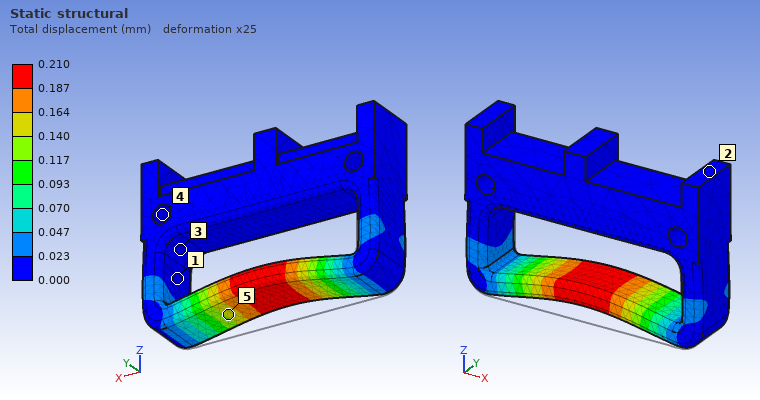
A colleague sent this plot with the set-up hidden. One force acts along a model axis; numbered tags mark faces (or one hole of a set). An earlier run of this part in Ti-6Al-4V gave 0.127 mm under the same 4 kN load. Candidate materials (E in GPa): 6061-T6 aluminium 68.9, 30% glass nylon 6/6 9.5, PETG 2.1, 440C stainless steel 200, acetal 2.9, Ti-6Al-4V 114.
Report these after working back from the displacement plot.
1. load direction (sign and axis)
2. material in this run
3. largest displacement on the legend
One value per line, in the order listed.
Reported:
+Z
6061-T6 aluminium
0.210 mm
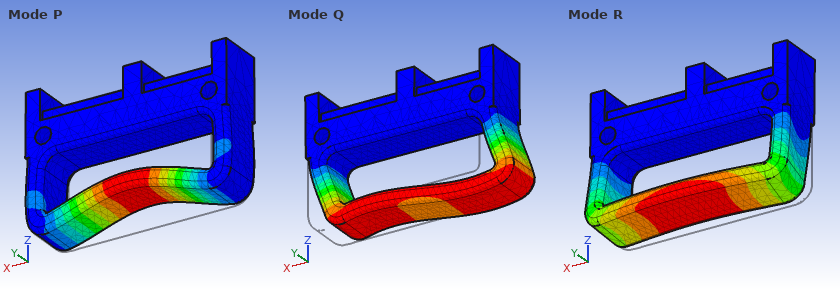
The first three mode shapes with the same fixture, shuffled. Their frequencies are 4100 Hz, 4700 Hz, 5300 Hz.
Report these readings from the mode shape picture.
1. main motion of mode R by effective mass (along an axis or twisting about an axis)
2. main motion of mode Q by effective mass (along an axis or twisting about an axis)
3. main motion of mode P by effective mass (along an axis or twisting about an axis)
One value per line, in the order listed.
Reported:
along Y
along X
along Z
